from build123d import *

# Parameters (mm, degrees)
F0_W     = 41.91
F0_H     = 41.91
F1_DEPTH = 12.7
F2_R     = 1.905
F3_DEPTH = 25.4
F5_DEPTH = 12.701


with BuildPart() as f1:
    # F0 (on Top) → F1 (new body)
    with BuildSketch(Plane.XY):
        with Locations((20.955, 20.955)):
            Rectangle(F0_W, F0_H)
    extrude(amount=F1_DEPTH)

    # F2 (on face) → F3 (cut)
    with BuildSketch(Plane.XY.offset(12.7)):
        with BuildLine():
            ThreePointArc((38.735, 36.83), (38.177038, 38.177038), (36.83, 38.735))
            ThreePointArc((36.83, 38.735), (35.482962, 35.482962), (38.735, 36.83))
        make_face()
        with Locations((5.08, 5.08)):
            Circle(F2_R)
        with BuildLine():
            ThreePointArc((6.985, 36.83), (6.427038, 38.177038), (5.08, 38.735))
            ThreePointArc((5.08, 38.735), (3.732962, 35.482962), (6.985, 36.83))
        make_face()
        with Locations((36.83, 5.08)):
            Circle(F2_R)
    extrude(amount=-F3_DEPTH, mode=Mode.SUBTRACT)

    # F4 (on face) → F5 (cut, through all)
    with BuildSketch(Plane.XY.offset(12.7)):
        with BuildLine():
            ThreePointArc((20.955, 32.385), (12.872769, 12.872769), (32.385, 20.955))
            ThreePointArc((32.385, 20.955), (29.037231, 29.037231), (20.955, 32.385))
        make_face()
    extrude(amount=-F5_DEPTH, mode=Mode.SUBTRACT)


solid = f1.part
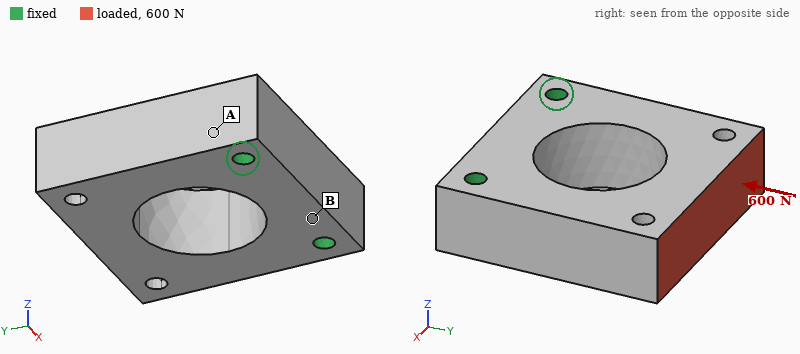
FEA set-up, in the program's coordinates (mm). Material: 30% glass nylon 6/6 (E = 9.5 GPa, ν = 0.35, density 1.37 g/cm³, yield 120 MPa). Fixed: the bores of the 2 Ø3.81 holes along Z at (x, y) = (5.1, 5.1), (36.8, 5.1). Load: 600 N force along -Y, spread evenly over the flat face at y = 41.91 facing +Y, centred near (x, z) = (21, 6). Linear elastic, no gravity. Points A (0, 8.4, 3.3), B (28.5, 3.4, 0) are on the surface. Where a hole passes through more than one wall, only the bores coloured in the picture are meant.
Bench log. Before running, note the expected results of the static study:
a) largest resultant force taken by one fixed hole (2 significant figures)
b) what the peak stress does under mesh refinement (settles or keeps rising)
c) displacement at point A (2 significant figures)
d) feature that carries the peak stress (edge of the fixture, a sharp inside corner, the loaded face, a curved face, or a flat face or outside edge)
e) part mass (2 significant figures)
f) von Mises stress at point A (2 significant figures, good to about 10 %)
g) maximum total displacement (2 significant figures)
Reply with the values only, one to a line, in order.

300 N
keeps rising
2.2 µm
edge of the fixture
23 g
2.1 MPa
14 µm
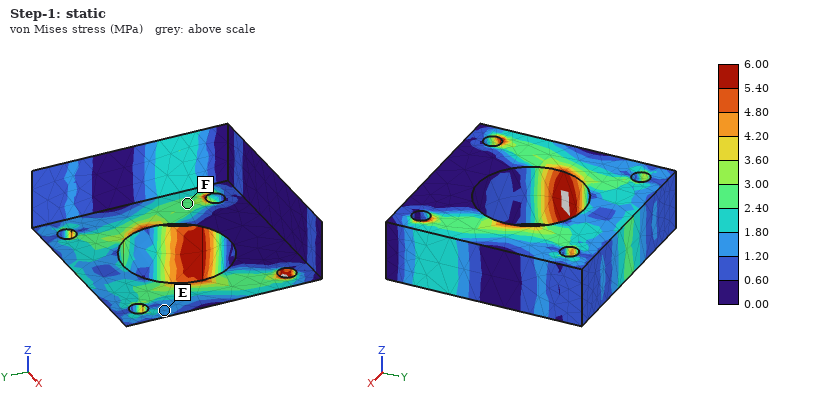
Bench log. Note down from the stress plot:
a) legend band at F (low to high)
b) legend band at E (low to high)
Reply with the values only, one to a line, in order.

2.40 to 3.00 MPa
1.20 to 1.80 MPa
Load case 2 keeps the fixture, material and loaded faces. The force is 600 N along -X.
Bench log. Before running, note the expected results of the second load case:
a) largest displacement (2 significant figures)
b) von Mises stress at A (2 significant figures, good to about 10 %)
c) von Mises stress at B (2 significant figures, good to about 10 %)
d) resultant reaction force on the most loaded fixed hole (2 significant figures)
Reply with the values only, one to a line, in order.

81 µm
9.6 MPa
2.6 MPa
670 N
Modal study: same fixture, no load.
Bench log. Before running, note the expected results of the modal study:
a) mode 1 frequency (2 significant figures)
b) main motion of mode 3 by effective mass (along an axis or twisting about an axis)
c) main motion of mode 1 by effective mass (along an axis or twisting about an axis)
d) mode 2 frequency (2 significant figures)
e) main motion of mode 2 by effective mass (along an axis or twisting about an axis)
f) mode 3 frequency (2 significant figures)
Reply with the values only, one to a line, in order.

2900 Hz
twisting about Y
along Z
4800 Hz
along X
5700 Hz
